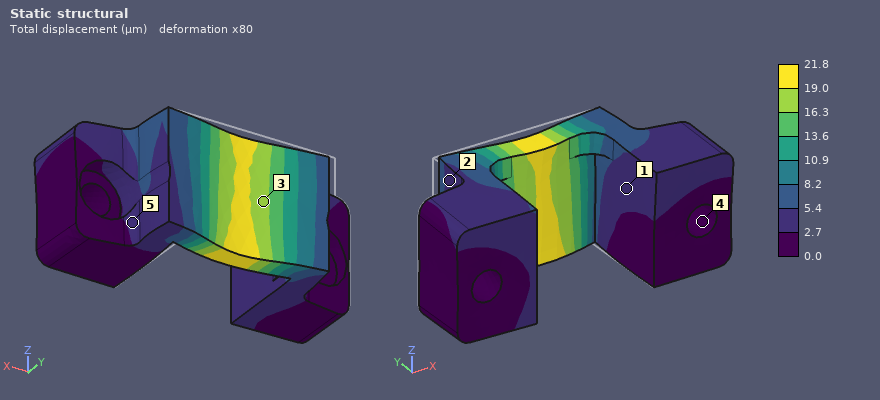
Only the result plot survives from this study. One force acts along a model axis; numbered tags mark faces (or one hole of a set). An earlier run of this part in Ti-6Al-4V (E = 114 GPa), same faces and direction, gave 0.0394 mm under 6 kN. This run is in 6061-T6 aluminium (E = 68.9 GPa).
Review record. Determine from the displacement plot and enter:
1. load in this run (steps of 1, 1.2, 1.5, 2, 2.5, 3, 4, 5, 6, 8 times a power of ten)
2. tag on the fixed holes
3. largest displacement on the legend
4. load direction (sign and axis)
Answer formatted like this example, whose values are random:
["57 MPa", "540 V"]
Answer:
["2 kN", "4", "21.8 µm", "-Y"]
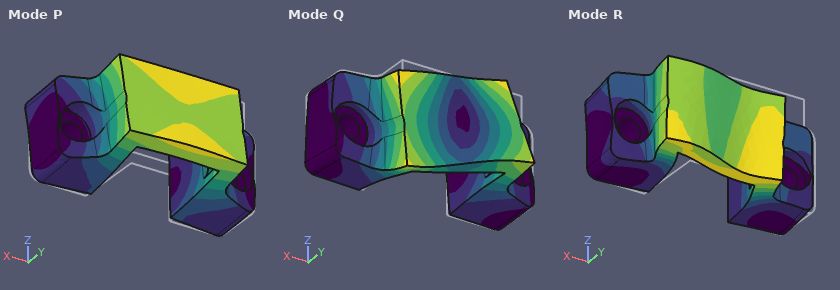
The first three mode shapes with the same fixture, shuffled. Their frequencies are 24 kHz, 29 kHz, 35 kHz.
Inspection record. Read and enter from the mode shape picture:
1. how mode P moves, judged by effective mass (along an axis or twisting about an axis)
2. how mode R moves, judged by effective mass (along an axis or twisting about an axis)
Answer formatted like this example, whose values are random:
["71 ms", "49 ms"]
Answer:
["along Z", "along X"]
